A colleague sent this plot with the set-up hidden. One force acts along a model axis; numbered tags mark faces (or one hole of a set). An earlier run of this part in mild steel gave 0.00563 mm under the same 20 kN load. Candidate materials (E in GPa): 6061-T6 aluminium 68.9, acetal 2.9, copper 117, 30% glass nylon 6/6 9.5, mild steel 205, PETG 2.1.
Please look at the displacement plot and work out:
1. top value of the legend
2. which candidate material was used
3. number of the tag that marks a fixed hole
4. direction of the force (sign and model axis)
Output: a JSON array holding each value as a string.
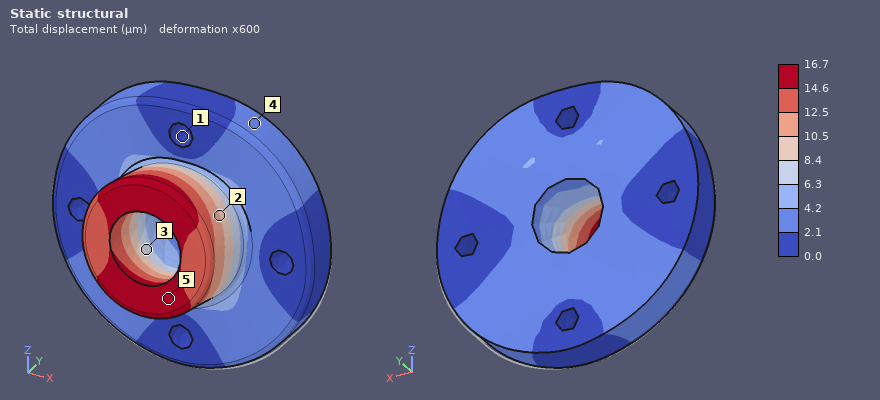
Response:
["16.7 µm", "6061-T6 aluminium", "1", "+Z"]
